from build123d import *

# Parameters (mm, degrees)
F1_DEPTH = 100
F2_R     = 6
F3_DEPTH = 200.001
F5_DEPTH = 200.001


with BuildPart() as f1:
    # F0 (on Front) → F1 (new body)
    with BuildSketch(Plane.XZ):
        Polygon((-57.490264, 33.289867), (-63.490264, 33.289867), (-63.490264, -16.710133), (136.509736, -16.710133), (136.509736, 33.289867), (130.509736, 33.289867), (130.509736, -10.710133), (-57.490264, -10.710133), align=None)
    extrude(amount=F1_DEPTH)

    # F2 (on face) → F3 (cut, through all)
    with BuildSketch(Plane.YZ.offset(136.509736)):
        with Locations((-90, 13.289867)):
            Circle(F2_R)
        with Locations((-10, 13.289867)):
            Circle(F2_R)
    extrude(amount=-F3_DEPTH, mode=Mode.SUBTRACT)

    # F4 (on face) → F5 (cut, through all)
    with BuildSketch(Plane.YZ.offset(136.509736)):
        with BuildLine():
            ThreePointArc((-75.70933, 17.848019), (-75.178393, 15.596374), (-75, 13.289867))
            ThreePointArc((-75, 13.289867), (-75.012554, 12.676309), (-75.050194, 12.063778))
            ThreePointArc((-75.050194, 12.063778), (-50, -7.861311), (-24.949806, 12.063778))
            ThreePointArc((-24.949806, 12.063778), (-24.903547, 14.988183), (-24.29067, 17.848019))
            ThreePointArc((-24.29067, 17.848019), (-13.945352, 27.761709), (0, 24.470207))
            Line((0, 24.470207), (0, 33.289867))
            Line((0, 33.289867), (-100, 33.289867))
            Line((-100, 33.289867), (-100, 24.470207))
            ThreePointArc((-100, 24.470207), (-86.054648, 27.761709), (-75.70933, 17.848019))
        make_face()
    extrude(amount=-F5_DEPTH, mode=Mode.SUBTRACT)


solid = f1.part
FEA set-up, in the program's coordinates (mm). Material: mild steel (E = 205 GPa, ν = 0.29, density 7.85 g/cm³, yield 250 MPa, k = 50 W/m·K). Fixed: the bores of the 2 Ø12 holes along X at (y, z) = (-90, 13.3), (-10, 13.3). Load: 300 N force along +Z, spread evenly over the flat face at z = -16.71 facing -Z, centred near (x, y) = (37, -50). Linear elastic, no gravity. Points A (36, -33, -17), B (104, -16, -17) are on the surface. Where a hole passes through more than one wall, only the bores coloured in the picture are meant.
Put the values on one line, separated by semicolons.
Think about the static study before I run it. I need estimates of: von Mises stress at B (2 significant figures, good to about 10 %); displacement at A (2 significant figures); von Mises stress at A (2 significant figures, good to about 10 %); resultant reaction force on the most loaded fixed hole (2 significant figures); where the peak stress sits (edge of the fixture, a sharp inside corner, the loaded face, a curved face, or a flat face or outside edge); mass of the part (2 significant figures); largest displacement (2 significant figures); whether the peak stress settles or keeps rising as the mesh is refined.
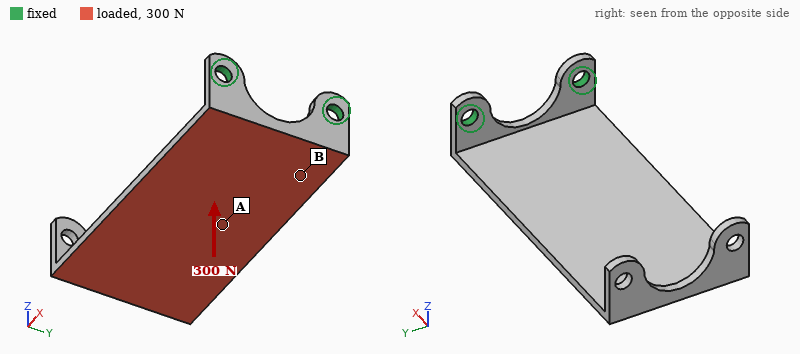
34 MPa; 0.53 mm; 12 MPa; 170 N; edge of the fixture; 1.1 kg; 1.3 mm; keeps rising
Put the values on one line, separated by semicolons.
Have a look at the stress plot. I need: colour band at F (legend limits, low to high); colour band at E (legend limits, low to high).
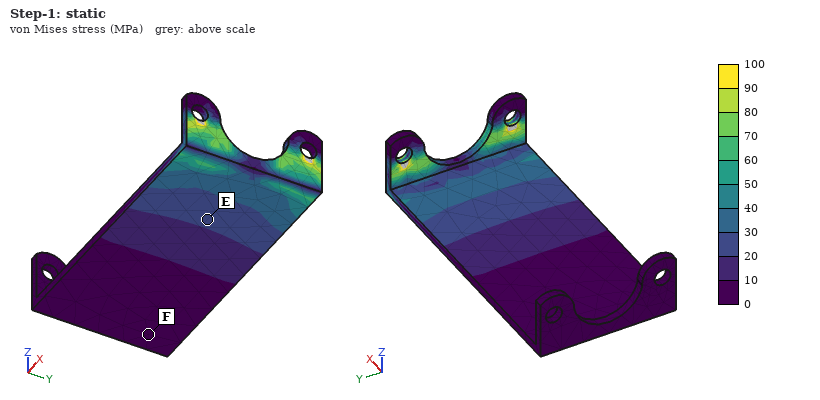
0 to 10 MPa; 20 to 30 MPa
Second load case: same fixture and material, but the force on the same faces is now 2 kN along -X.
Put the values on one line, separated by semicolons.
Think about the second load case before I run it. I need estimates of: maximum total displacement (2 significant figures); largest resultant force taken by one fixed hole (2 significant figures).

0.80 mm; 1.0 kN
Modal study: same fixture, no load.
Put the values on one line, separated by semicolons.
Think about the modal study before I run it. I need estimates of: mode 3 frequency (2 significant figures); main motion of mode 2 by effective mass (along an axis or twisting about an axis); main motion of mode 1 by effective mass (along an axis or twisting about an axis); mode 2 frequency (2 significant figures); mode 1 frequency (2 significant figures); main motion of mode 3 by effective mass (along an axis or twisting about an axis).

530 Hz; along Y; along Z; 370 Hz; 85 Hz; along Y
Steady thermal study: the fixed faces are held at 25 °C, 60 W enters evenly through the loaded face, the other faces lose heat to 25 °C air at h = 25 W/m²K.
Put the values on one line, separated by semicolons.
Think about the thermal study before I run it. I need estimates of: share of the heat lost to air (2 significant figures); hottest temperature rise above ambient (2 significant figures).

68 %; 67 K
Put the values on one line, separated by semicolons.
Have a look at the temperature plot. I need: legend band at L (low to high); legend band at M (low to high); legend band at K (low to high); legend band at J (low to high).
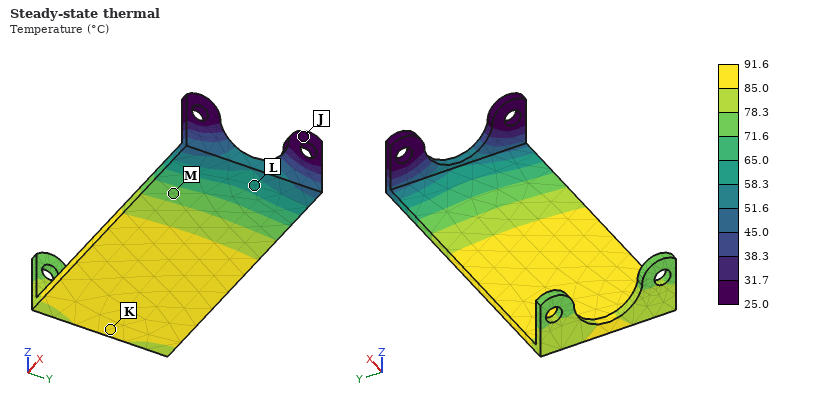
58.3 to 65.0 °C; 71.6 to 78.3 °C; 85.0 to 91.6 °C; 25.0 to 31.7 °C
